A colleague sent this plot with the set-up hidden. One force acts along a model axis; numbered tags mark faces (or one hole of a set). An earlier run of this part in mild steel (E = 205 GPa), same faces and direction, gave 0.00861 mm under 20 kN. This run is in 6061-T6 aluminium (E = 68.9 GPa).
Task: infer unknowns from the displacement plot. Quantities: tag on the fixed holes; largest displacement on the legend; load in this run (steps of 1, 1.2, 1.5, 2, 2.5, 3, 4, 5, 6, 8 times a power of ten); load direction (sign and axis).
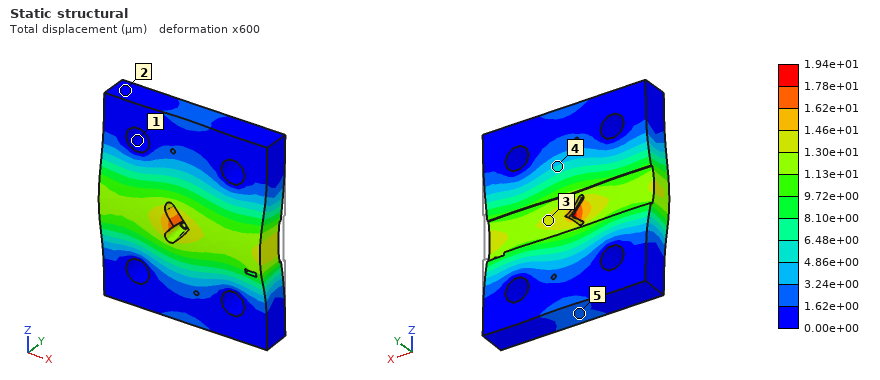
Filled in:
1
1.94e+01 µm
15 kN
-Y
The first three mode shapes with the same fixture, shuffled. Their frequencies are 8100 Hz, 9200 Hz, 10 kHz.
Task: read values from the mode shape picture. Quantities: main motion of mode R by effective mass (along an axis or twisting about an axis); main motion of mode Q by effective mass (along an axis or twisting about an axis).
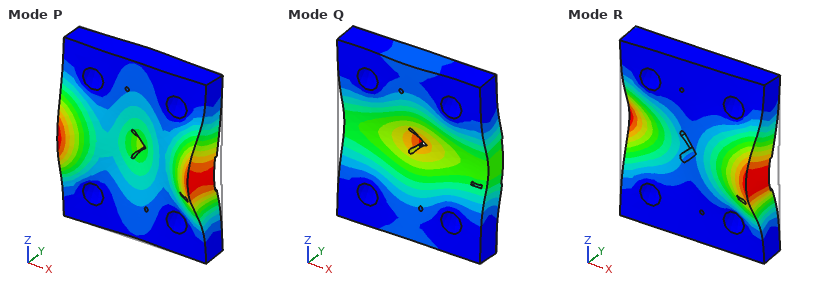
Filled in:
twisting about Z
along Y
